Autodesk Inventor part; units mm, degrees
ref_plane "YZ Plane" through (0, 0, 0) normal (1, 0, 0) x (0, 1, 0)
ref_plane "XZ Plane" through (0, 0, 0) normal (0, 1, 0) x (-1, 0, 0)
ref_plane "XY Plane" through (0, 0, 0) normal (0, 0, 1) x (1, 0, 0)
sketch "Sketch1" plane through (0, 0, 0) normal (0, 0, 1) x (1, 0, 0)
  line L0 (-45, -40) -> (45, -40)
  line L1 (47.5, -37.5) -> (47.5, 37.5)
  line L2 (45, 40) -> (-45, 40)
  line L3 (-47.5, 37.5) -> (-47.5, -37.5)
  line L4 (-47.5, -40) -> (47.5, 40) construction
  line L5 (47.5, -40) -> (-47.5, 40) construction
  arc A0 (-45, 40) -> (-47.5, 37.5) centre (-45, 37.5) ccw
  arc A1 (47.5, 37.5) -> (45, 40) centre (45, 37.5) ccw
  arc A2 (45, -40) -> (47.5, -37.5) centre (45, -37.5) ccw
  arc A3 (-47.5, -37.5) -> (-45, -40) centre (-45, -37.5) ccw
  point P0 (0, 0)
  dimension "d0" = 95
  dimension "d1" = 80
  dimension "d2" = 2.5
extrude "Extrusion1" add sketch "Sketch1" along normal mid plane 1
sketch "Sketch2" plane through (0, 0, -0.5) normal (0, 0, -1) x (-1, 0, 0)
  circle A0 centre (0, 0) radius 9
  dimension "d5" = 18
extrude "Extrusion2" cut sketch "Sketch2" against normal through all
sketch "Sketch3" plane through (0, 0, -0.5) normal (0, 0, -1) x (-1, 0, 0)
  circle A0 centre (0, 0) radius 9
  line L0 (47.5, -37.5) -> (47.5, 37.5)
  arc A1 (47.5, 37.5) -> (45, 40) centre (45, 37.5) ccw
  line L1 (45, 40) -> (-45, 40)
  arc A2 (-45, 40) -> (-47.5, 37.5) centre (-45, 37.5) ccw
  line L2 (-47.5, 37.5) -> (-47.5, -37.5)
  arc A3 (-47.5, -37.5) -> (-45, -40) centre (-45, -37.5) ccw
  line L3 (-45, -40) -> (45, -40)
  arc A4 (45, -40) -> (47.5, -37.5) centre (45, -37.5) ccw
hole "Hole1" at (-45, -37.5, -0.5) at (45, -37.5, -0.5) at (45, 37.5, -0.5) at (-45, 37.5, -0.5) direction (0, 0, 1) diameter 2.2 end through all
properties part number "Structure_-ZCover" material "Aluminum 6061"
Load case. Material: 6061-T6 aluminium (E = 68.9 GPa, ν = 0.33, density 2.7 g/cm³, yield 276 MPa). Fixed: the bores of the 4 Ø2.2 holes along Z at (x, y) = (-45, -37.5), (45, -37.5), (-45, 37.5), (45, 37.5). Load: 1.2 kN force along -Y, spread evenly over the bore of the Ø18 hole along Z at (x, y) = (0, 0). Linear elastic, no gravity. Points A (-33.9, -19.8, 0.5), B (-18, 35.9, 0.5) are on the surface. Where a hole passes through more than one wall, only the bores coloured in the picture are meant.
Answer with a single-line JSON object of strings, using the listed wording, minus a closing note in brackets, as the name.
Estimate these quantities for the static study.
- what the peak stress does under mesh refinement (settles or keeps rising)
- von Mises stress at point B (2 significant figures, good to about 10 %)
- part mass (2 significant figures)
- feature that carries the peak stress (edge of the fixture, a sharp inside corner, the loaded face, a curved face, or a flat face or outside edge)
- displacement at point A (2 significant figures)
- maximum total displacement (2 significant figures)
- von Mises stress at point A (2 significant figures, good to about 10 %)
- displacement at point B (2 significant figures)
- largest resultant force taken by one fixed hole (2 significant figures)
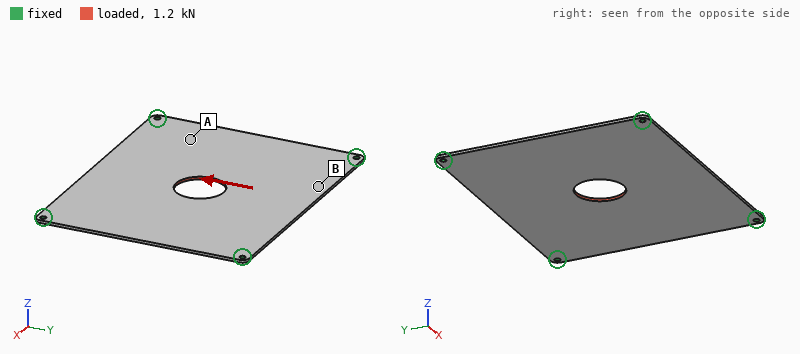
{"what the peak stress does under mesh refinement": "keeps rising", "von Mises stress at point B": "6.2 MPa", "part mass": "20 g", "feature that carries the peak stress": "edge of the fixture", "displacement at point A": "9.7 µm", "maximum total displacement": "23 µm", "von Mises stress at point A": "16 MPa", "displacement at point B": "16 µm", "largest resultant force taken by one fixed hole": "360 N"}
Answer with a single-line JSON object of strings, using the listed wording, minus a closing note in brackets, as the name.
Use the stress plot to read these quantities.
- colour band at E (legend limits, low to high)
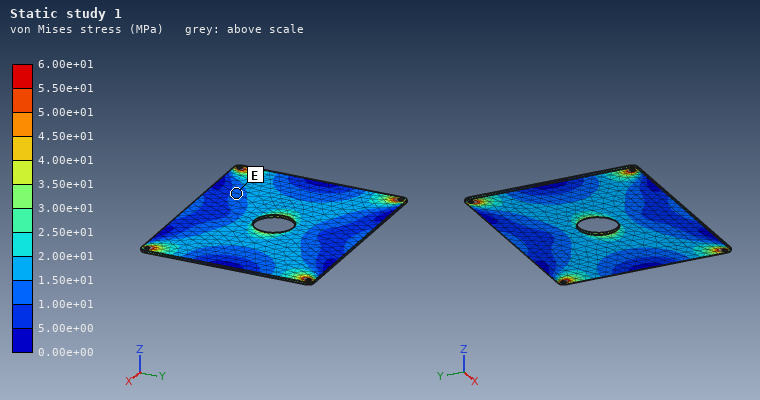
{"colour band at E": "1.00e+01 to 1.50e+01 MPa"}
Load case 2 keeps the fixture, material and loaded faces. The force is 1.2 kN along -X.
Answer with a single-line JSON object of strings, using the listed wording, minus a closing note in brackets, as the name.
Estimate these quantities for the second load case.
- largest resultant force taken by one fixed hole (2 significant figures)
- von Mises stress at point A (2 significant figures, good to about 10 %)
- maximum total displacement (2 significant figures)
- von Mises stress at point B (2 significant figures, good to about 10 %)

{"largest resultant force taken by one fixed hole": "340 N", "von Mises stress at point A": "12 MPa", "maximum total displacement": "18 µm", "von Mises stress at point B": "8.6 MPa"}
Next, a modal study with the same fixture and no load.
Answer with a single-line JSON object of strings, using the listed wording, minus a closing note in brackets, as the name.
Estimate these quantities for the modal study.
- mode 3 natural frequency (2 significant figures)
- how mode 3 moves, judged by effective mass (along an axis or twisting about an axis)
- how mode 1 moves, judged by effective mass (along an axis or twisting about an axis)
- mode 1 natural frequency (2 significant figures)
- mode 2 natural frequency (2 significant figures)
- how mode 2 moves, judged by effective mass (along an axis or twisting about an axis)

{"mode 3 natural frequency": "890 Hz", "how mode 3 moves, judged by effective mass": "twisting about Y", "how mode 1 moves, judged by effective mass": "along Z", "mode 1 natural frequency": "420 Hz", "mode 2 natural frequency": "750 Hz", "how mode 2 moves, judged by effective mass": "twisting about X"}
